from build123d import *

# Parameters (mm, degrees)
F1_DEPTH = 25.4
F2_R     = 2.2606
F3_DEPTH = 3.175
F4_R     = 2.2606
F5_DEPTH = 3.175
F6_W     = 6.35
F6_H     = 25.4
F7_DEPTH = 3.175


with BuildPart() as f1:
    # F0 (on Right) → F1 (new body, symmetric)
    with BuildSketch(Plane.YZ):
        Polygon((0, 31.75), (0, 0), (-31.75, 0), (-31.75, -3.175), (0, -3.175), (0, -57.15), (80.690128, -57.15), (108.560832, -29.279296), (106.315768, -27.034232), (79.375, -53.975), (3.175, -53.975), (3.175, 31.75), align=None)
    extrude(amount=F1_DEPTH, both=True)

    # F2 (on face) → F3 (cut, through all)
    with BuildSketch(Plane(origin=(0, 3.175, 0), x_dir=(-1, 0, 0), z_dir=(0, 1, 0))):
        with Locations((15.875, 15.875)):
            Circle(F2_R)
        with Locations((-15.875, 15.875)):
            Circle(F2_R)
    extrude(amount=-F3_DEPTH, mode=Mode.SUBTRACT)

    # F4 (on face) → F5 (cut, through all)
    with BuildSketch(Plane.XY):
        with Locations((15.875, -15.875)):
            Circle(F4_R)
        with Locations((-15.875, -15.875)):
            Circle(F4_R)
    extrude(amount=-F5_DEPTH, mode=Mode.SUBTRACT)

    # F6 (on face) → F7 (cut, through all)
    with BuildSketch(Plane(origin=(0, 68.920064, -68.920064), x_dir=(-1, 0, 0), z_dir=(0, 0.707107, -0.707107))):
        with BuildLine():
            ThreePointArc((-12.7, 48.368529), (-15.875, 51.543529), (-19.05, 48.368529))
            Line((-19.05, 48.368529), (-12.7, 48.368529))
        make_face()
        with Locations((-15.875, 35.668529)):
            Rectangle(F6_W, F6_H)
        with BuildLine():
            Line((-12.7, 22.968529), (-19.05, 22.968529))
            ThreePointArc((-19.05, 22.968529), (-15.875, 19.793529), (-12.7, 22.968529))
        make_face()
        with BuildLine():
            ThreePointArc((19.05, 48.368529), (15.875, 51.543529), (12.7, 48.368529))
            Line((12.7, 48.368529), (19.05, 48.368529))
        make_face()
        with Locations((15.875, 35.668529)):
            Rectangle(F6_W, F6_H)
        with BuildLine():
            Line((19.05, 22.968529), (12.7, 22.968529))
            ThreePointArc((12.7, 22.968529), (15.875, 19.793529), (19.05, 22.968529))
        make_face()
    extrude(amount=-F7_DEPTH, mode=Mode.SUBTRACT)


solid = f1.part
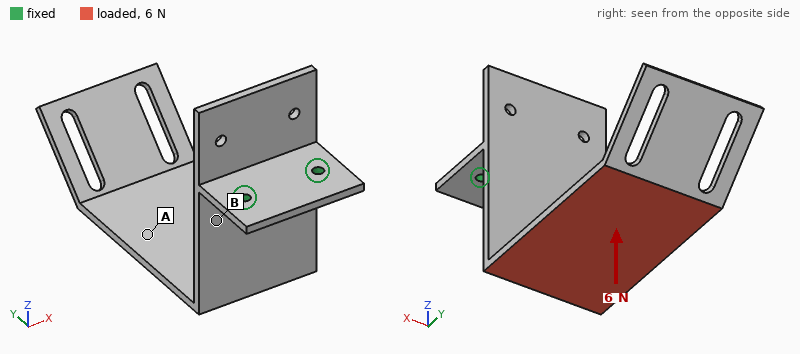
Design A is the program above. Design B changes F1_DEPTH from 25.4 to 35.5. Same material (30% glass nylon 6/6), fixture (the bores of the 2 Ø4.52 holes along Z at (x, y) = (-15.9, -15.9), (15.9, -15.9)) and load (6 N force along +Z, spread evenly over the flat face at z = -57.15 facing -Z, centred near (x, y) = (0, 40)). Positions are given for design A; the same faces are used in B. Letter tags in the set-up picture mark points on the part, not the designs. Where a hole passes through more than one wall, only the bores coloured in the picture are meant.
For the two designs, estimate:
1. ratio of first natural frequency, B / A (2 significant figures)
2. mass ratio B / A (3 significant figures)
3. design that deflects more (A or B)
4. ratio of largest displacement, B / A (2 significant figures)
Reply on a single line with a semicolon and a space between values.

0.97; 1.41; A; 0.72
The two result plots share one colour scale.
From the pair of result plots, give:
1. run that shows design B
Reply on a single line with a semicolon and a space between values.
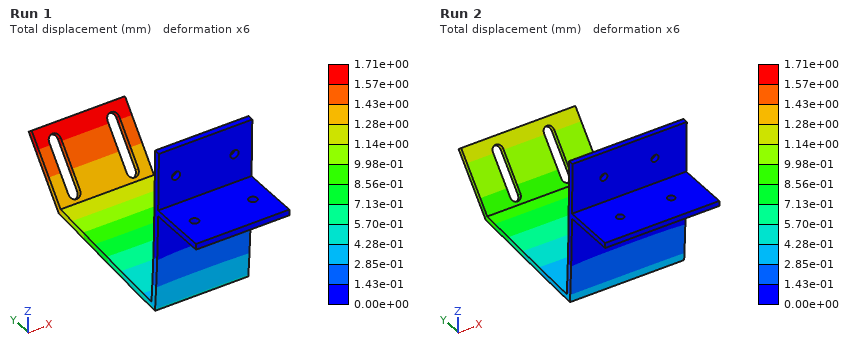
Run 2
